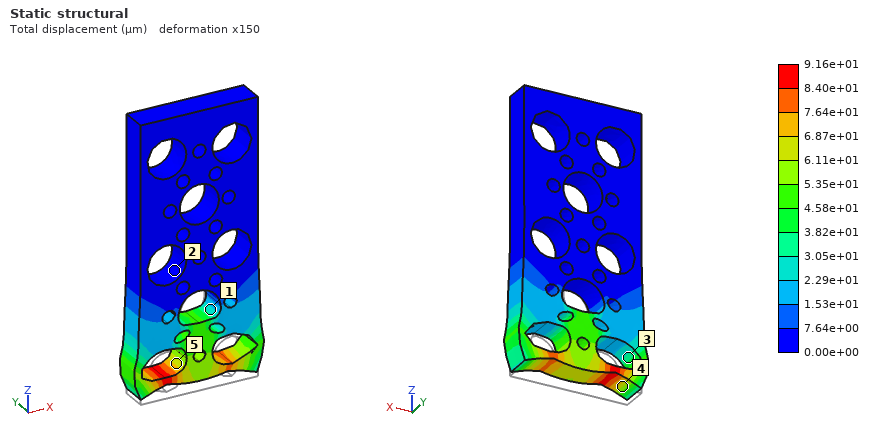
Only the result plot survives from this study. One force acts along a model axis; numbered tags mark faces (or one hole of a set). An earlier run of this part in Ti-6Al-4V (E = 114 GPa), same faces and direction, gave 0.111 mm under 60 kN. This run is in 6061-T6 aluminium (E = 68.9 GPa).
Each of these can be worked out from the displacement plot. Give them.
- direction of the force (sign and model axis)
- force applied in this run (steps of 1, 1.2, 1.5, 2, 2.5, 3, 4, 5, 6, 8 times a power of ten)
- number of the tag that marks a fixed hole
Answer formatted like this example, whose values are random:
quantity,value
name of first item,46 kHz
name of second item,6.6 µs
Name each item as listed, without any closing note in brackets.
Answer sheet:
quantity,value
direction of the force,+Z
force applied in this run,30 kN
number of the tag that marks a fixed hole,2
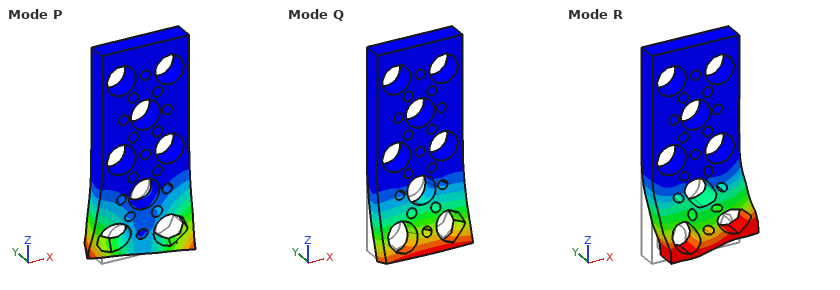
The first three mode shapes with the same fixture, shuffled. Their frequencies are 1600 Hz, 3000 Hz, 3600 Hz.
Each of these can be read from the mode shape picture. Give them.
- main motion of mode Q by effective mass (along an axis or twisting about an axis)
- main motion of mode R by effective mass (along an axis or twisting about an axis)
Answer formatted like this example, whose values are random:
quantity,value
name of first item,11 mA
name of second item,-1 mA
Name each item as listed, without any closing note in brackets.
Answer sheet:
quantity,value
main motion of mode Q by effective mass,along Y
main motion of mode R by effective mass,along X
